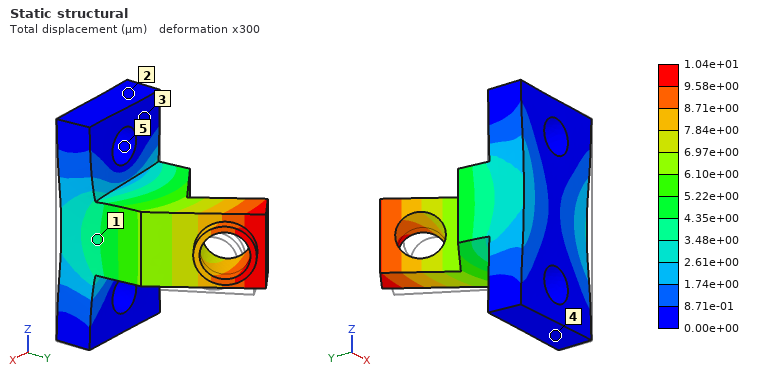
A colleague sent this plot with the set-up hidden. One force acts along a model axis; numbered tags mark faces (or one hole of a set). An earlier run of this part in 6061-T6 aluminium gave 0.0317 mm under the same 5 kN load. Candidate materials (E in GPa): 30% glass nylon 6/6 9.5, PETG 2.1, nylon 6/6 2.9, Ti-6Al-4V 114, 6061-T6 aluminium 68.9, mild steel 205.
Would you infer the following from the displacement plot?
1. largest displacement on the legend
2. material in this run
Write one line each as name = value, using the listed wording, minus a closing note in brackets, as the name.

largest displacement on the legend = 1.04e+01 µm
material in this run = mild steel
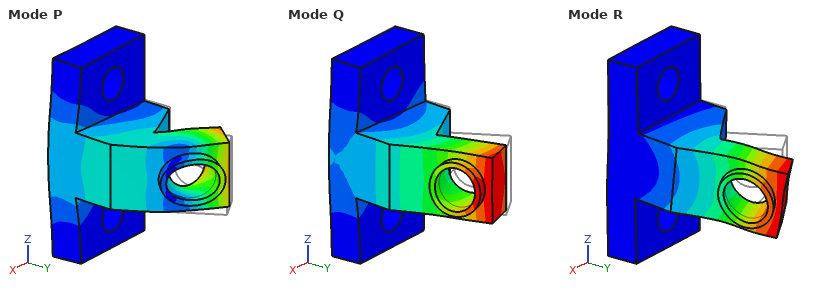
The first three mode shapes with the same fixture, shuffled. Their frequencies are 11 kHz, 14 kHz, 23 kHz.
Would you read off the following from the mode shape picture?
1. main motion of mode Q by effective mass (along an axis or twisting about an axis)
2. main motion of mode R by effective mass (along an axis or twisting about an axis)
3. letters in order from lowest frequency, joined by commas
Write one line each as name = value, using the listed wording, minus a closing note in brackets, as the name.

main motion of mode Q by effective mass = along X
main motion of mode R by effective mass = along Z
letters in order from lowest frequency, joined by commas = Q, R, P
